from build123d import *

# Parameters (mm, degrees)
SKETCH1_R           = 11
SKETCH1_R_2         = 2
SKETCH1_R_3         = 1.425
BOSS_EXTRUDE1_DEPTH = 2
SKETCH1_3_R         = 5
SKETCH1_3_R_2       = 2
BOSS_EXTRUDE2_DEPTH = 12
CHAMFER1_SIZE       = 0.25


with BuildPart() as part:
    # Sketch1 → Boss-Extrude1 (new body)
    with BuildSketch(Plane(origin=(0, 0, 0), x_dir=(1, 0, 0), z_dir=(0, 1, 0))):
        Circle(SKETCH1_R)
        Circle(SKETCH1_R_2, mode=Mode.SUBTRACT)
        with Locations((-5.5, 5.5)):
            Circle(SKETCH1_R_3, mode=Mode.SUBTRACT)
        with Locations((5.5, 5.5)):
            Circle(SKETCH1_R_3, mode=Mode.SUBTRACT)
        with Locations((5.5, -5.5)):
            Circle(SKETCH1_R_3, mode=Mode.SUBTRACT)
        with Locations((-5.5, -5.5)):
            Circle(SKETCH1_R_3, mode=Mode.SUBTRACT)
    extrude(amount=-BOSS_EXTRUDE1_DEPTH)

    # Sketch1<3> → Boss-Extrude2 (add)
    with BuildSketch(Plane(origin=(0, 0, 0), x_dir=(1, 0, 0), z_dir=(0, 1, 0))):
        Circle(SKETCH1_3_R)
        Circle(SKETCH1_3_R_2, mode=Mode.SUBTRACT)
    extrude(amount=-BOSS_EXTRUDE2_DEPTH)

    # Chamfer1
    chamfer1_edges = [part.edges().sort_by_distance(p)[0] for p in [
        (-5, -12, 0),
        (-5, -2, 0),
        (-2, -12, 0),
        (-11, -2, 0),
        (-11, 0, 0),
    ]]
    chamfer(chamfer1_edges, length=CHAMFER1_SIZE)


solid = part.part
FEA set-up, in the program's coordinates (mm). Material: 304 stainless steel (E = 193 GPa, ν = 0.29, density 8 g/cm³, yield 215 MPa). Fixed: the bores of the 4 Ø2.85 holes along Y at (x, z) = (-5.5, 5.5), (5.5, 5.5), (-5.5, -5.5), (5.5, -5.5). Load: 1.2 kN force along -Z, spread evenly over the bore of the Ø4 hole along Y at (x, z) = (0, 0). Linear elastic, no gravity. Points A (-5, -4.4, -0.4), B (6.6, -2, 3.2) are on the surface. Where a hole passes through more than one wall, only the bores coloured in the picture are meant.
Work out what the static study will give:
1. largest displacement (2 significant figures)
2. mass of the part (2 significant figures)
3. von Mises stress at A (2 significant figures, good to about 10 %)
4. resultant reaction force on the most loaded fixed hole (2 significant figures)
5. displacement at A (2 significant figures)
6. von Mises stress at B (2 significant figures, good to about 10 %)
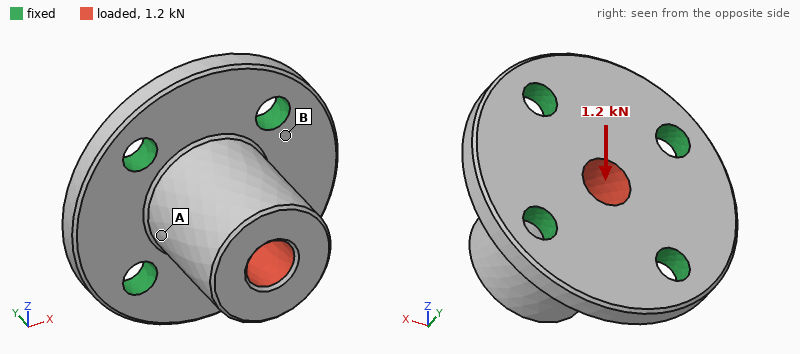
7.4 µm
11 g
23 MPa
450 N
2.1 µm
12 MPa
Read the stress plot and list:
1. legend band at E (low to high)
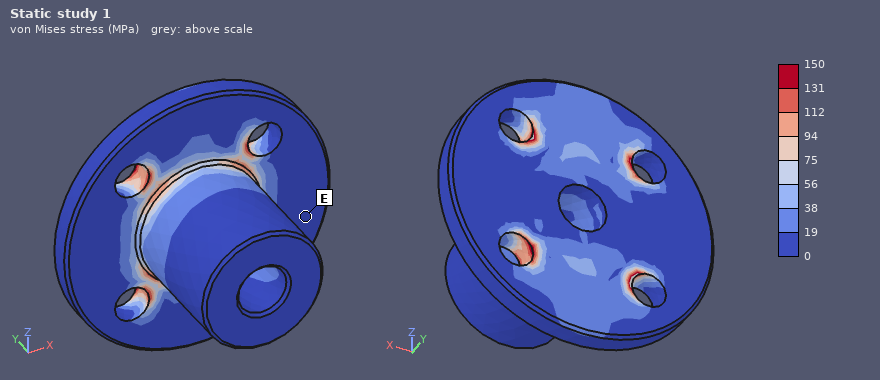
0 to 19 MPa
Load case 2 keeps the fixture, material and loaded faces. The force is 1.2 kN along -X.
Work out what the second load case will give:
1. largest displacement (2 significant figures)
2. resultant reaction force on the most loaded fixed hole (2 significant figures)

7.5 µm
450 N
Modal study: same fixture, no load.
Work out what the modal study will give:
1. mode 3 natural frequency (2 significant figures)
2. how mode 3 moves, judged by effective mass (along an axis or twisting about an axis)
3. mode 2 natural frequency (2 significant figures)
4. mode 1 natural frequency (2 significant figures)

49 kHz
along Y
29 kHz
29 kHz
